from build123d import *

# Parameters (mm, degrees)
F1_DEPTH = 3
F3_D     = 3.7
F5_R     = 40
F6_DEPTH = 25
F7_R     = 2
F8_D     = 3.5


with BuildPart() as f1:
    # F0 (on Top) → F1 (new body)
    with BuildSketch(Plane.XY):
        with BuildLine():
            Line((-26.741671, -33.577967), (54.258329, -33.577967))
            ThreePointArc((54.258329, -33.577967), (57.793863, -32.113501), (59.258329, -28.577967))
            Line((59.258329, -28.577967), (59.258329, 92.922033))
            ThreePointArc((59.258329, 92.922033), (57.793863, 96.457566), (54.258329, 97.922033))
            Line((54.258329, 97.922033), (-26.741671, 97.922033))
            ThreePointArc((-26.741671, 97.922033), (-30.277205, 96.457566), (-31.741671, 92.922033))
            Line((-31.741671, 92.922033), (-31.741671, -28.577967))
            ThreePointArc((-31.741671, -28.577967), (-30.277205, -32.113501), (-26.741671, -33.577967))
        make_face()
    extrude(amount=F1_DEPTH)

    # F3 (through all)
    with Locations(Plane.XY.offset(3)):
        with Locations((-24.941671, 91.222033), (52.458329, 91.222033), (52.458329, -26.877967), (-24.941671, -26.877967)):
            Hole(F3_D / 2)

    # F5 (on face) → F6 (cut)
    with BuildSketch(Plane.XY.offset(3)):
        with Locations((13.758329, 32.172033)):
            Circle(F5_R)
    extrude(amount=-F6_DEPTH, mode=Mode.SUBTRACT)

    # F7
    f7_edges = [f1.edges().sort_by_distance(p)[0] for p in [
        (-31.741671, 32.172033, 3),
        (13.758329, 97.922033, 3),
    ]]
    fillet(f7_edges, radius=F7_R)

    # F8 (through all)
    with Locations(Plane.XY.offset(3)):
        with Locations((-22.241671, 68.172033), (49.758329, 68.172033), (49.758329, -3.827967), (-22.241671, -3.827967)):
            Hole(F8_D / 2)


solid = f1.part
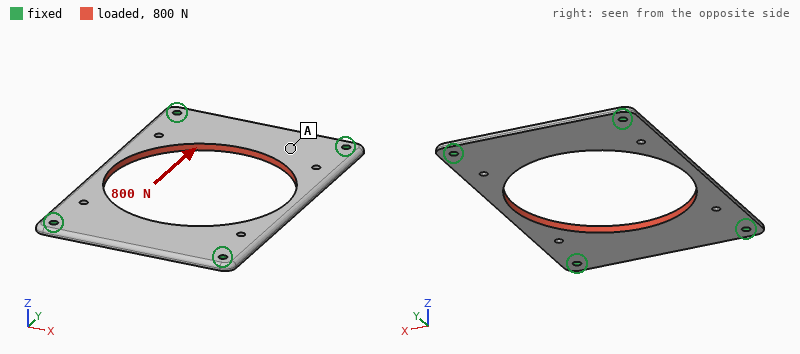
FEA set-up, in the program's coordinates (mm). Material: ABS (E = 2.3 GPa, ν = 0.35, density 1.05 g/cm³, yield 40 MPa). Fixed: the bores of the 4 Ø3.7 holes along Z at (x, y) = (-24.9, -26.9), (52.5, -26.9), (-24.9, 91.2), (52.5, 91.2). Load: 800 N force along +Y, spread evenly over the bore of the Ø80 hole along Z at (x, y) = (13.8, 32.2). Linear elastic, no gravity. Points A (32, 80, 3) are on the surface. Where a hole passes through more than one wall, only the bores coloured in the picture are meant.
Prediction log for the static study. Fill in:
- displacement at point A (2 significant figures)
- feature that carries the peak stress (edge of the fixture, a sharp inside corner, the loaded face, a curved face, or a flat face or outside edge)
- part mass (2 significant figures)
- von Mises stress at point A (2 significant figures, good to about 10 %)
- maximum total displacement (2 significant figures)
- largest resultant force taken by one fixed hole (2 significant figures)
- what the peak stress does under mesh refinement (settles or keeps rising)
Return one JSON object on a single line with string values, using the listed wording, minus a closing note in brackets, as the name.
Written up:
{"displacement at point A": "0.082 mm", "feature that carries the peak stress": "edge of the fixture", "part mass": "21 g", "von Mises stress at point A": "2.3 MPa", "maximum total displacement": "0.11 mm", "largest resultant force taken by one fixed hole": "210 N", "what the peak stress does under mesh refinement": "keeps rising"}
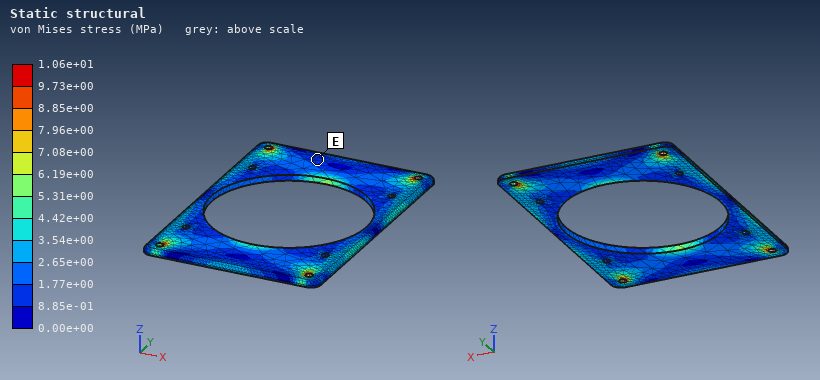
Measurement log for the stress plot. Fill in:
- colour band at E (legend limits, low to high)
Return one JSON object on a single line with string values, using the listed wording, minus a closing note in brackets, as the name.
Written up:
{"colour band at E": "8.85e-01 to 1.77e+00 MPa"}
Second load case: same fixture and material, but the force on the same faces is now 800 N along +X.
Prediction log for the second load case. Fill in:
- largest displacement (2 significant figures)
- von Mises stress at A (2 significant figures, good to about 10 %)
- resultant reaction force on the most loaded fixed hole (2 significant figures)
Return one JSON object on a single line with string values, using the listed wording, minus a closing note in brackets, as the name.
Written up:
{"largest displacement": "0.46 mm", "von Mises stress at A": "3.7 MPa", "resultant reaction force on the most loaded fixed hole": "210 N"}
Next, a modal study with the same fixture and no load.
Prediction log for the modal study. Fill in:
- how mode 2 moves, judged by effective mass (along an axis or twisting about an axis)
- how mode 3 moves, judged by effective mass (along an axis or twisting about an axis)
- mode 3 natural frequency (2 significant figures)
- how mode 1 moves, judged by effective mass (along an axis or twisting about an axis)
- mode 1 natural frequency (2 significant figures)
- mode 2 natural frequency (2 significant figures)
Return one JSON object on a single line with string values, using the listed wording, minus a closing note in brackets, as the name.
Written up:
{"how mode 2 moves, judged by effective mass": "twisting about Y", "how mode 3 moves, judged by effective mass": "twisting about X", "mode 3 natural frequency": "630 Hz", "how mode 1 moves, judged by effective mass": "along Z", "mode 1 natural frequency": "400 Hz", "mode 2 natural frequency": "460 Hz"}
